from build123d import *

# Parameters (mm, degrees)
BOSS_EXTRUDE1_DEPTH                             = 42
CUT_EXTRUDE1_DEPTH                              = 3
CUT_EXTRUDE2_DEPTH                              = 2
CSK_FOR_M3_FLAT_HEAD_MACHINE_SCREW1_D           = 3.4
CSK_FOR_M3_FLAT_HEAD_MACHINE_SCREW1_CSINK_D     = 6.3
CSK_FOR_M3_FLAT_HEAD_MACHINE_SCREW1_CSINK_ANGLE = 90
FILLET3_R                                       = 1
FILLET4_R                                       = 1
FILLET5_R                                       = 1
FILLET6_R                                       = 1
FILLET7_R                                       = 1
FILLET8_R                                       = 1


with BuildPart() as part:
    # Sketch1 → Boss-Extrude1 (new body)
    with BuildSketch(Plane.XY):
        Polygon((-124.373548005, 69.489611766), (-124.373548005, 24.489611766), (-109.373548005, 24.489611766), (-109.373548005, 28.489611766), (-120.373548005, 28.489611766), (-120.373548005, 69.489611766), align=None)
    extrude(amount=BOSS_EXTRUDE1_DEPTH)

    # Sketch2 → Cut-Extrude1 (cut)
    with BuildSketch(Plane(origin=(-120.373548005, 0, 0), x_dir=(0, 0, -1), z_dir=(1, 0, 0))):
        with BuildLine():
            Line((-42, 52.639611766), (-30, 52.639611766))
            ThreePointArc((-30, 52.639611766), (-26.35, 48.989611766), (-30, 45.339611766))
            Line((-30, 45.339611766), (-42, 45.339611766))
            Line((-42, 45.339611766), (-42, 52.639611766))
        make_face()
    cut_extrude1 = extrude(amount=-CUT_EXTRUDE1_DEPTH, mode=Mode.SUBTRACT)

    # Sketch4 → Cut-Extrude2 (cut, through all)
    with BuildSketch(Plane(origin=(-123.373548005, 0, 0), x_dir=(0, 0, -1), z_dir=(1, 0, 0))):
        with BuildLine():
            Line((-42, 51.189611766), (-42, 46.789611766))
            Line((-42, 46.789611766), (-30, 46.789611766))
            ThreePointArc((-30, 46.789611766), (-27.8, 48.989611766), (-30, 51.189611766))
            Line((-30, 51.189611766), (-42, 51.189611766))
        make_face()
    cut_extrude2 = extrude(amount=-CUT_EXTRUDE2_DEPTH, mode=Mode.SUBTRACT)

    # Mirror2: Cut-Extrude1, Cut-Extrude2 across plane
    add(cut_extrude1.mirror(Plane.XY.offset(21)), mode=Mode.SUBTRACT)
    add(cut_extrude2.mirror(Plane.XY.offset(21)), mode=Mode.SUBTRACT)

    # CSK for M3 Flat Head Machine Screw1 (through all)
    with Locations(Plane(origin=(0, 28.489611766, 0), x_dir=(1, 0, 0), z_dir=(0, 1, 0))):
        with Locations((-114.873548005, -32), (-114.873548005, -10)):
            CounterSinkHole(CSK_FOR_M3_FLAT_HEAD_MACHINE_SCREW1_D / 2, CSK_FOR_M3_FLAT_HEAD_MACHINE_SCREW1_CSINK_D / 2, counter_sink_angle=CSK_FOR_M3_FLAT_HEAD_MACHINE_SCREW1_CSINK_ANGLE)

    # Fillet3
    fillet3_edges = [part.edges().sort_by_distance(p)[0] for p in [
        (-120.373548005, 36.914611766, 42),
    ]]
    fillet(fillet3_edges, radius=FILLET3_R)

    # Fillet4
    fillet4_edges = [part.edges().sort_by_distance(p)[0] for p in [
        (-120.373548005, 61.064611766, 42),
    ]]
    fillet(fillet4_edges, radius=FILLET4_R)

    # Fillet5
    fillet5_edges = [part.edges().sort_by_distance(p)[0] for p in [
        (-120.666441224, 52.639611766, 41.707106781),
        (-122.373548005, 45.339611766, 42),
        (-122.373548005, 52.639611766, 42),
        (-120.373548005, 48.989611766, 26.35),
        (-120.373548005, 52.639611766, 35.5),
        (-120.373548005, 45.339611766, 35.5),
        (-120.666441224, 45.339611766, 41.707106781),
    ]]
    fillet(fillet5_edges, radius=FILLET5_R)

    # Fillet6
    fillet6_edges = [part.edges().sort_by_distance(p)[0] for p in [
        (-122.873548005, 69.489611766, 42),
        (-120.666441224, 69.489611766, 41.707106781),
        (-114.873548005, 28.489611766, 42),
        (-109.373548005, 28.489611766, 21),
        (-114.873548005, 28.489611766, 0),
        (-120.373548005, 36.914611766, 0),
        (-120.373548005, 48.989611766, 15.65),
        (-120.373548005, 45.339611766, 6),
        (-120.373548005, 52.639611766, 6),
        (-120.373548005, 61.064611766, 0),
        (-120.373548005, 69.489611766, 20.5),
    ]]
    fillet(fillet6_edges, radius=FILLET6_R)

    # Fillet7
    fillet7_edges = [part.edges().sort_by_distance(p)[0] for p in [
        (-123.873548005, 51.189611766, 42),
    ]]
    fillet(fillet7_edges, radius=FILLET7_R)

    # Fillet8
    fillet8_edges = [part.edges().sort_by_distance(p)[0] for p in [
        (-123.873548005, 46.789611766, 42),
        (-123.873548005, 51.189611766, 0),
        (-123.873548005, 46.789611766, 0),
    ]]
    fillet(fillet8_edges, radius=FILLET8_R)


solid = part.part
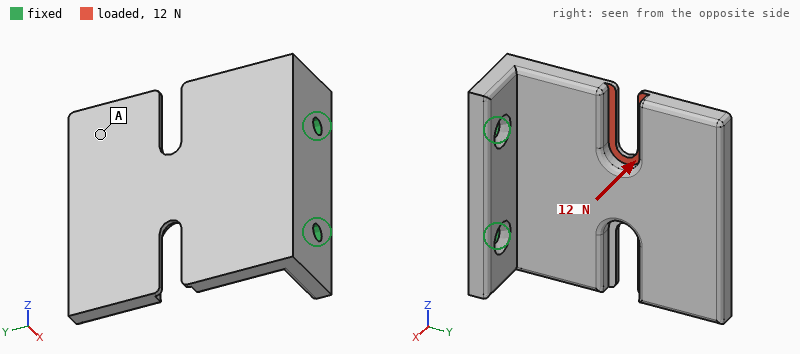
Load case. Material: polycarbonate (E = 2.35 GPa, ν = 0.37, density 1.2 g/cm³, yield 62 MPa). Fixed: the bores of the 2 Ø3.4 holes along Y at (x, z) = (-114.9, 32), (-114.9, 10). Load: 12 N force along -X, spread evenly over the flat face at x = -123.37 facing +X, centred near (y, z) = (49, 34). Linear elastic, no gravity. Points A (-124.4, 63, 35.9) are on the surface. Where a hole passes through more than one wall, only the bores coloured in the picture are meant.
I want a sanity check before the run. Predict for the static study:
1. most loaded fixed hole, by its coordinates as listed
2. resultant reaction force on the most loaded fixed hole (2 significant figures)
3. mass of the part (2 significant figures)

(-114.9, 32)
13 N
10 g
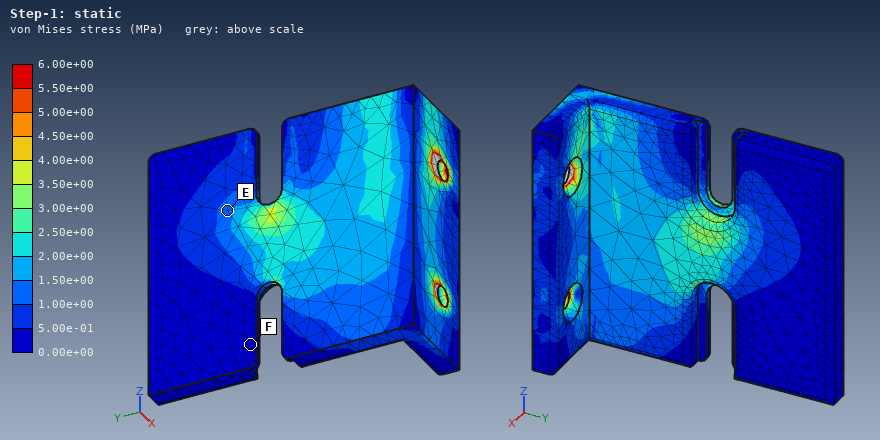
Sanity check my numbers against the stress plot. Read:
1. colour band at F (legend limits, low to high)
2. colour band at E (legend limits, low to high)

0.00e+00 to 5.00e-01 MPa
1.00e+00 to 1.50e+00 MPa
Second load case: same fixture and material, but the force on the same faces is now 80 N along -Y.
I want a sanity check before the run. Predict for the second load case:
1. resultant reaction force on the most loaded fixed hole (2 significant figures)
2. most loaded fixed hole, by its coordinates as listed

82 N
(-114.9, 32)
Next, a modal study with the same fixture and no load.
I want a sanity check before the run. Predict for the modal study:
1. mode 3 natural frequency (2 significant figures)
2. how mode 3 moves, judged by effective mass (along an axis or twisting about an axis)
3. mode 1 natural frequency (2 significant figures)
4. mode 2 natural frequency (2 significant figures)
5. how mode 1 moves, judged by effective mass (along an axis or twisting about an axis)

1000 Hz
along Z
330 Hz
700 Hz
along X
